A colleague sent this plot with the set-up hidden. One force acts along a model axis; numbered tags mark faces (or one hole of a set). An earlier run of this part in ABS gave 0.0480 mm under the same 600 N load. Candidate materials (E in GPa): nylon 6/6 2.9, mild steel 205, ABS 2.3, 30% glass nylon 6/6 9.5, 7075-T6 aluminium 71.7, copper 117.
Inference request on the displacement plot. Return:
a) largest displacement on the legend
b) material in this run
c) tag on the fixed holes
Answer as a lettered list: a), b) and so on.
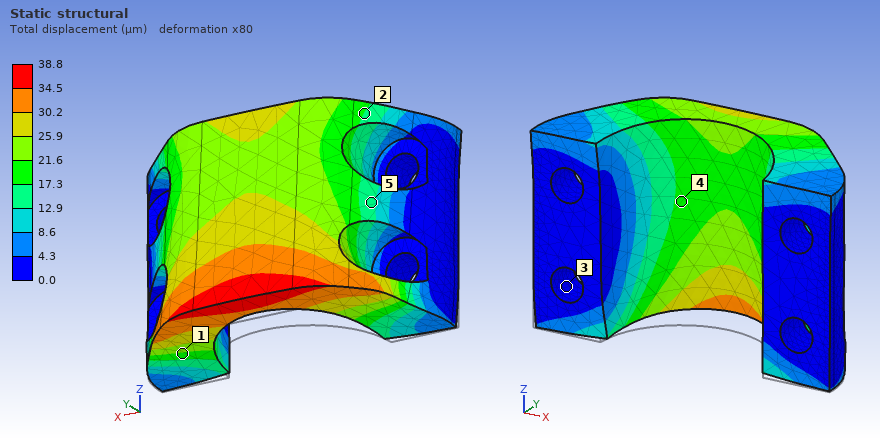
a) 38.8 µm
b) nylon 6/6
c) 3
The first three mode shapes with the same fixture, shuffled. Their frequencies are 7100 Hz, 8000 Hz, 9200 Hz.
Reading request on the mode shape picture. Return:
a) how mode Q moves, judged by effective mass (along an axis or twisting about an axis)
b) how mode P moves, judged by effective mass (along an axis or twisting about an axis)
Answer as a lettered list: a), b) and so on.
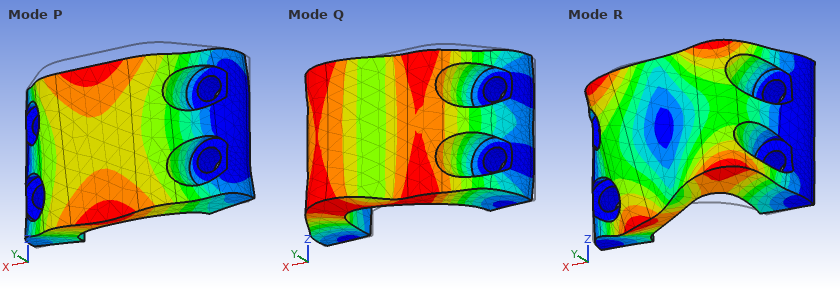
a) along X
b) along Z
